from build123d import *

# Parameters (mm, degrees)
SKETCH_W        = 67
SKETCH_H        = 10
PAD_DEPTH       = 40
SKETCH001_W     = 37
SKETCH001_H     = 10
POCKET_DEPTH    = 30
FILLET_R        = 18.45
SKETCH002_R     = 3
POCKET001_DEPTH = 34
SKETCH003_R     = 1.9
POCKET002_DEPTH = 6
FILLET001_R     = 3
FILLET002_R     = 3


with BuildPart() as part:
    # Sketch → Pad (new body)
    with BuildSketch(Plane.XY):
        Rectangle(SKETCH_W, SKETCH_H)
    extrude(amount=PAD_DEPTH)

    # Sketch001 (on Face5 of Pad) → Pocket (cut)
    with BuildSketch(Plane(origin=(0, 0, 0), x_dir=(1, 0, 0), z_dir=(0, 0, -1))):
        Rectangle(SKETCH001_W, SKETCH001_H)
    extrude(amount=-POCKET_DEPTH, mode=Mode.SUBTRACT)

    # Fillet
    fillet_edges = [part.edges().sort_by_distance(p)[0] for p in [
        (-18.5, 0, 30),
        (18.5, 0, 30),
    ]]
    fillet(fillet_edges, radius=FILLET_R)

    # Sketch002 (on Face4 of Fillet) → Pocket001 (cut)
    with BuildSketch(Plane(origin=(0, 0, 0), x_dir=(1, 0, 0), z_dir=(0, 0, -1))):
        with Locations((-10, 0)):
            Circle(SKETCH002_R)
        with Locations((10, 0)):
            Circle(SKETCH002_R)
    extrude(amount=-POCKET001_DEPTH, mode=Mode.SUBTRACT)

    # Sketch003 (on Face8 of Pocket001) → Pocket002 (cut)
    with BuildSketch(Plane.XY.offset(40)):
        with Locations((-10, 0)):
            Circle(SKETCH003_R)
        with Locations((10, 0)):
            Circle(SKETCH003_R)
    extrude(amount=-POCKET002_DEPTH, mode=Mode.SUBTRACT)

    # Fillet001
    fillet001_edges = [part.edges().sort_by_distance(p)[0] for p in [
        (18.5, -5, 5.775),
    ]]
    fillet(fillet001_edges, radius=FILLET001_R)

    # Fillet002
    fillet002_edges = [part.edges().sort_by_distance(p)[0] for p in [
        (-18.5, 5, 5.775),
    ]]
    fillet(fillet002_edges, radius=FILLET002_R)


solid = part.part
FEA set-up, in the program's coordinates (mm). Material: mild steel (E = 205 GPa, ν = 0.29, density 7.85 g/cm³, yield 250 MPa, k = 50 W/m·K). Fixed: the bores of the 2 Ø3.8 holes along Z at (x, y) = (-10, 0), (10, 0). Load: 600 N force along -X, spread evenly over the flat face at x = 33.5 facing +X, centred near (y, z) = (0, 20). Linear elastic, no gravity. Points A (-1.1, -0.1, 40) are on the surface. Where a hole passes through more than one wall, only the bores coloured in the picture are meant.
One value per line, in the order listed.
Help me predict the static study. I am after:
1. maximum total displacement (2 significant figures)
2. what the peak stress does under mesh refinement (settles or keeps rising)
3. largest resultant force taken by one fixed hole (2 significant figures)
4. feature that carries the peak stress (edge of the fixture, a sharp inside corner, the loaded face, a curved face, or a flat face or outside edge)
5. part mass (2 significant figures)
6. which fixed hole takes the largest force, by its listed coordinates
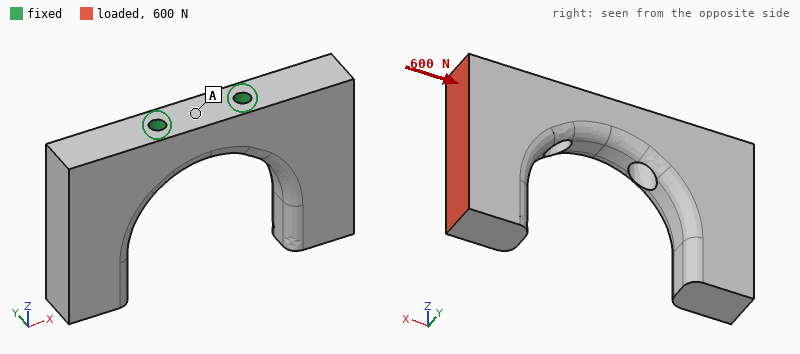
22 µm
keeps rising
480 N
edge of the fixture
130 g
(-10, 0)
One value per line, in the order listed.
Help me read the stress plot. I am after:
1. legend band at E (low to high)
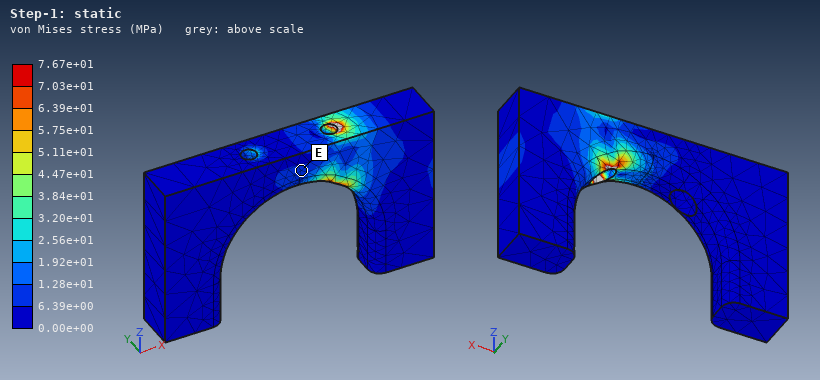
6.39e+00 to 1.28e+01 MPa
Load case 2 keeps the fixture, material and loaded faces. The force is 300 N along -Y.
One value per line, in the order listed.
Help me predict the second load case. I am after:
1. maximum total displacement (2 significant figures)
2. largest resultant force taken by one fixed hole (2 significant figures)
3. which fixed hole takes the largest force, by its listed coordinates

27 µm
480 N
(10, 0)
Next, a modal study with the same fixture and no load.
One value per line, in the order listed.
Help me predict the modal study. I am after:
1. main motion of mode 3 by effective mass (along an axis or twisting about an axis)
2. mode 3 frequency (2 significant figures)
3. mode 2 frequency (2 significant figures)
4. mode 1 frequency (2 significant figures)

along Z
4100 Hz
3400 Hz
3400 Hz
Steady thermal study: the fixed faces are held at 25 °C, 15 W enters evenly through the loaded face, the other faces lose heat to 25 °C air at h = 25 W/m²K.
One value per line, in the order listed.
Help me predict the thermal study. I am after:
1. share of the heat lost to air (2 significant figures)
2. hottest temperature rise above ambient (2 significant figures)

13 %
52 K
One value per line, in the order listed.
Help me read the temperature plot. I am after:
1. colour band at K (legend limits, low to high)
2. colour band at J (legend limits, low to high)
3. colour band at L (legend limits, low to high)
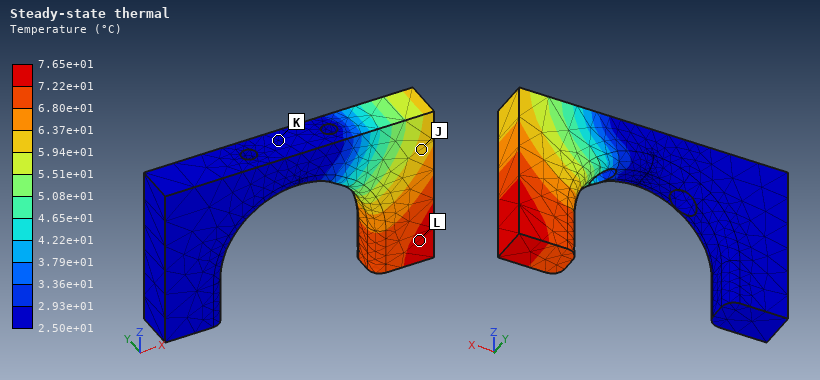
2.50e+01 to 2.93e+01 °C
5.94e+01 to 6.37e+01 °C
7.22e+01 to 7.65e+01 °C
